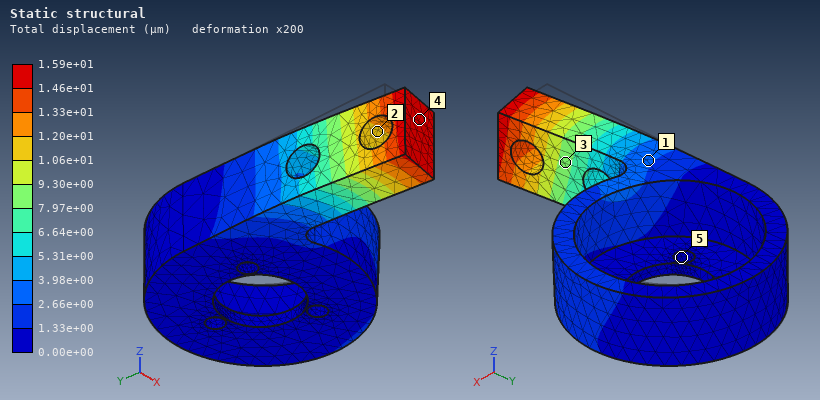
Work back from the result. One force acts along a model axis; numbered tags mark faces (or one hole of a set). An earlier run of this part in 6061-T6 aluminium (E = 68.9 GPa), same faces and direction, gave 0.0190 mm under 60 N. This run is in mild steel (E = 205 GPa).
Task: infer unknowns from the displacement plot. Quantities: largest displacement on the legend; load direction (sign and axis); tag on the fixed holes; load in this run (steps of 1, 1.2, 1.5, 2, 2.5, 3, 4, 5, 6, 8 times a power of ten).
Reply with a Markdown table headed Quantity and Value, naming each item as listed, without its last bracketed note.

| Quantity | Value |
|---|---|
| largest displacement on the legend | 1.59e+01 µm |
| load direction | +X |
| tag on the fixed holes | 5 |
| load in this run | 150 N |
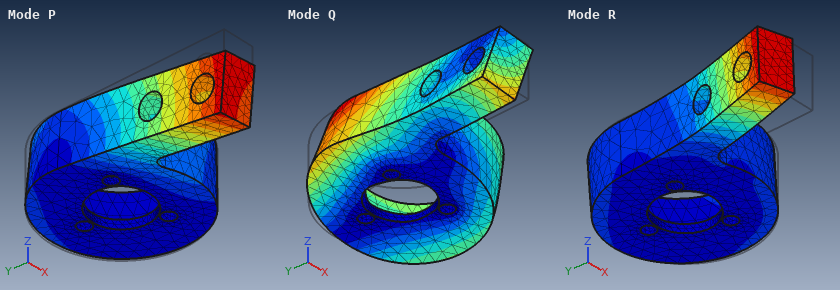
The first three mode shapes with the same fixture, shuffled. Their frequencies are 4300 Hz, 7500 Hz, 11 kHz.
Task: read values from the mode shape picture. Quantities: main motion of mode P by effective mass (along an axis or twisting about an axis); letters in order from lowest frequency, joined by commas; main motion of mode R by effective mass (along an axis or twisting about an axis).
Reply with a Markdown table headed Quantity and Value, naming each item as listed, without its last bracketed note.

| Quantity | Value |
|---|---|
| main motion of mode P by effective mass | along Z |
| letters in order from lowest frequency, joined by commas | P, R, Q |
| main motion of mode R by effective mass | along X |
